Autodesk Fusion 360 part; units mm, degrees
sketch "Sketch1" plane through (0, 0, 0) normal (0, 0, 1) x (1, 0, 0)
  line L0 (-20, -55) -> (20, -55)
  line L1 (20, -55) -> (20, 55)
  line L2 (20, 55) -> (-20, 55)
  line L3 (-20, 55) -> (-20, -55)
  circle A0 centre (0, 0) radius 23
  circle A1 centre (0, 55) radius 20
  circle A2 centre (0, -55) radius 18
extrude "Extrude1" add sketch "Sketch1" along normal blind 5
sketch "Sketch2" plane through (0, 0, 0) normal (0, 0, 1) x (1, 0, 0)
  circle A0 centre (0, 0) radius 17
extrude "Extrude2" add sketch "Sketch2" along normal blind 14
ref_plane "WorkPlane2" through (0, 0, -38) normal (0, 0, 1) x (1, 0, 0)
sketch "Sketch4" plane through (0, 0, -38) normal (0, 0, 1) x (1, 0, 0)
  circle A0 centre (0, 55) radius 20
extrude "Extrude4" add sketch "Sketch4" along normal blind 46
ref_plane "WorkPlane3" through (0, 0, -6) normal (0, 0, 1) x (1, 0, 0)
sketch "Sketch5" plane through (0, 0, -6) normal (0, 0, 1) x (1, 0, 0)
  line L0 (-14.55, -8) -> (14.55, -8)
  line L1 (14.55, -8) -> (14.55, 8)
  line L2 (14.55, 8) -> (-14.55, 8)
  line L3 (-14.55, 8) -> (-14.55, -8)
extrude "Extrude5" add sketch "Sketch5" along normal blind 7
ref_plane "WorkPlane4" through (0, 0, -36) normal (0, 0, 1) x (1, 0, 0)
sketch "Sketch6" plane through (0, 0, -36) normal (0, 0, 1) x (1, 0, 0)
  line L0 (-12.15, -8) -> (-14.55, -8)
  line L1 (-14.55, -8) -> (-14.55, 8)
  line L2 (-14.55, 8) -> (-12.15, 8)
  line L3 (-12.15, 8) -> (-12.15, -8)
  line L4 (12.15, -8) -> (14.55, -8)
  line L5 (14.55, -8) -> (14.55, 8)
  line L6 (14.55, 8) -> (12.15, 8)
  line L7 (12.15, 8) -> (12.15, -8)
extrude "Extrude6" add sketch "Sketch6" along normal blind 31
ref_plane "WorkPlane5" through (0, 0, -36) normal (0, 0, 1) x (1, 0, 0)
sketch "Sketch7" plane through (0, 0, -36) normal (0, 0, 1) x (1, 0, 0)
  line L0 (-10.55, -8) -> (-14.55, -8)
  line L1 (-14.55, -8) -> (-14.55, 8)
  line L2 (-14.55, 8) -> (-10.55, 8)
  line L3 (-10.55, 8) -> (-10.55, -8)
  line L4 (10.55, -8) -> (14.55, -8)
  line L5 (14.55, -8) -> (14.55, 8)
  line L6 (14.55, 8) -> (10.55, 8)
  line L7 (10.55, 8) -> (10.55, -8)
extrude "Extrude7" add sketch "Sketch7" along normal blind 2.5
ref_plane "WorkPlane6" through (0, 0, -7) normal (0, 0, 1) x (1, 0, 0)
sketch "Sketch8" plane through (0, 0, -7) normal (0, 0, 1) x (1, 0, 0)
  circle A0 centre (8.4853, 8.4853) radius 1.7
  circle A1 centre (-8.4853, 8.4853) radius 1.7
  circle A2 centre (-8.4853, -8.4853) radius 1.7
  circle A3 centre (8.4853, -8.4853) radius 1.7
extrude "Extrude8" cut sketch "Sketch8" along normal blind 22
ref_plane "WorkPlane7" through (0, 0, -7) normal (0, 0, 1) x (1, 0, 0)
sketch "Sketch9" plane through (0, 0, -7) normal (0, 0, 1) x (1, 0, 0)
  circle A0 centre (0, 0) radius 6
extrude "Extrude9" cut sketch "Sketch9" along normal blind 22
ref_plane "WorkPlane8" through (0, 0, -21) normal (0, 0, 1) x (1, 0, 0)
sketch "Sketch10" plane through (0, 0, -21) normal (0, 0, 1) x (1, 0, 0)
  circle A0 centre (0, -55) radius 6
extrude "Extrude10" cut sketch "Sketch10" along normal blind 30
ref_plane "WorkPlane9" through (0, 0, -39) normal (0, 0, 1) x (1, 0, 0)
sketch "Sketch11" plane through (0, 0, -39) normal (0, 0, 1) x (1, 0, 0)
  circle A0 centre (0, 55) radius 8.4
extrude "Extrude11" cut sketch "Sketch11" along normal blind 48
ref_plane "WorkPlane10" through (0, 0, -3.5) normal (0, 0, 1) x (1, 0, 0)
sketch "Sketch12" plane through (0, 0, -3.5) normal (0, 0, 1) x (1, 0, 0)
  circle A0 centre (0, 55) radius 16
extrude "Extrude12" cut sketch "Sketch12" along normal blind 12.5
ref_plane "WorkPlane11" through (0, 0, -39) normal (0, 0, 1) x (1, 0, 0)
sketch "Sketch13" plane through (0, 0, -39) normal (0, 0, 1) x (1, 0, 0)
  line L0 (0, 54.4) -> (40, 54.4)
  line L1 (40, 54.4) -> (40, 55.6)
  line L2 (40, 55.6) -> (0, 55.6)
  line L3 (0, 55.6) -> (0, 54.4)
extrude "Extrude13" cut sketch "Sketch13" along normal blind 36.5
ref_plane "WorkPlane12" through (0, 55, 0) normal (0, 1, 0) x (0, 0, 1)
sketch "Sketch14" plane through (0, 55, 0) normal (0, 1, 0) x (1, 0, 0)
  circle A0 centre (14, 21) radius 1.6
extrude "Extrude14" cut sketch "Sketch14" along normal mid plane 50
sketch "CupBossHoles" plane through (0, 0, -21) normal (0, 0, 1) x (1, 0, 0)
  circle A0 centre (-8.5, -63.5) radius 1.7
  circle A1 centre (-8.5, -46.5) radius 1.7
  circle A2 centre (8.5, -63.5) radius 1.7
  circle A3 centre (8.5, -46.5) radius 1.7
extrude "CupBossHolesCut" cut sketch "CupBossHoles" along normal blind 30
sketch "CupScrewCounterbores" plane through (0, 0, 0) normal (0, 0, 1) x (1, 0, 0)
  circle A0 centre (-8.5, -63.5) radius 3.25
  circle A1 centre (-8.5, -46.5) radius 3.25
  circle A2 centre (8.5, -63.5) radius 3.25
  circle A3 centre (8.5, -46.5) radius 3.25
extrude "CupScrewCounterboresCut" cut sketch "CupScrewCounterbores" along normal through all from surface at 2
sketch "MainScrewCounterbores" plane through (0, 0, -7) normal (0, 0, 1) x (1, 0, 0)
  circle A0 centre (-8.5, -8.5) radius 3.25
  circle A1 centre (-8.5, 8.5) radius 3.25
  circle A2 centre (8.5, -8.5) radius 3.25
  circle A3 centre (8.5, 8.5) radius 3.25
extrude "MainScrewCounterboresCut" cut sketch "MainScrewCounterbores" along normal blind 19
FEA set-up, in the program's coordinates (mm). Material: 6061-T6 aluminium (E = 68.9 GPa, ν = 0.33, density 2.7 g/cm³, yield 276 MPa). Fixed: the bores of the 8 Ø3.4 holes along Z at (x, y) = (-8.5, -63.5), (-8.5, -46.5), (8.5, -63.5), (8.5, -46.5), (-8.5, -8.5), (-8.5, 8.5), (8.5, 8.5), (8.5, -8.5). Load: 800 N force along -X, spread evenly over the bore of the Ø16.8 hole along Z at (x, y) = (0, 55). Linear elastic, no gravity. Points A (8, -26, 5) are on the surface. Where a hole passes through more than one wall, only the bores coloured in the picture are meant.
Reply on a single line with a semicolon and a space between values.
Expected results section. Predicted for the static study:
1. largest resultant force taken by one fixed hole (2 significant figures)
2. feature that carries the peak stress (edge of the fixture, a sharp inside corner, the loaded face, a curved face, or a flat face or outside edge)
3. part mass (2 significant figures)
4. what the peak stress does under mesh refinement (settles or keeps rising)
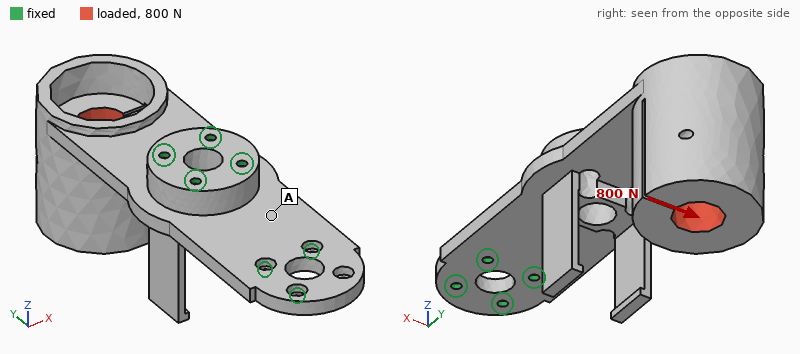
1.3 kN; edge of the fixture; 190 g; keeps rising
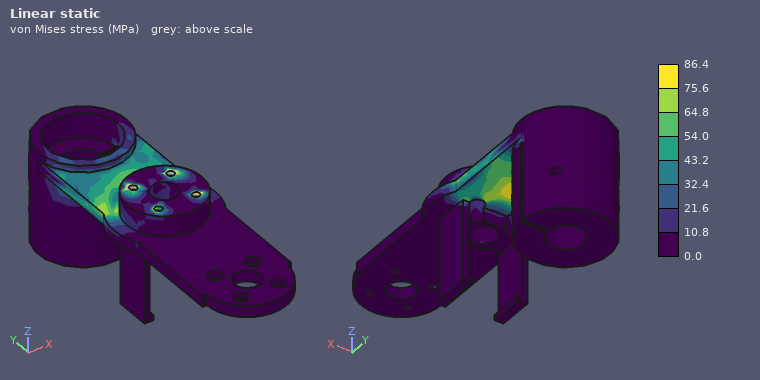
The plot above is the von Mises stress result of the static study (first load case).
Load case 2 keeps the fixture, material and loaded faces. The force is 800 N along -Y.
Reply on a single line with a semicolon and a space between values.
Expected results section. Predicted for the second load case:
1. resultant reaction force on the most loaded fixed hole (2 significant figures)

600 N
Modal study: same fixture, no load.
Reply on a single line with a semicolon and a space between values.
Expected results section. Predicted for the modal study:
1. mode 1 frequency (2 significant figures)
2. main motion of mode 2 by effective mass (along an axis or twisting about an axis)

390 Hz; along X
